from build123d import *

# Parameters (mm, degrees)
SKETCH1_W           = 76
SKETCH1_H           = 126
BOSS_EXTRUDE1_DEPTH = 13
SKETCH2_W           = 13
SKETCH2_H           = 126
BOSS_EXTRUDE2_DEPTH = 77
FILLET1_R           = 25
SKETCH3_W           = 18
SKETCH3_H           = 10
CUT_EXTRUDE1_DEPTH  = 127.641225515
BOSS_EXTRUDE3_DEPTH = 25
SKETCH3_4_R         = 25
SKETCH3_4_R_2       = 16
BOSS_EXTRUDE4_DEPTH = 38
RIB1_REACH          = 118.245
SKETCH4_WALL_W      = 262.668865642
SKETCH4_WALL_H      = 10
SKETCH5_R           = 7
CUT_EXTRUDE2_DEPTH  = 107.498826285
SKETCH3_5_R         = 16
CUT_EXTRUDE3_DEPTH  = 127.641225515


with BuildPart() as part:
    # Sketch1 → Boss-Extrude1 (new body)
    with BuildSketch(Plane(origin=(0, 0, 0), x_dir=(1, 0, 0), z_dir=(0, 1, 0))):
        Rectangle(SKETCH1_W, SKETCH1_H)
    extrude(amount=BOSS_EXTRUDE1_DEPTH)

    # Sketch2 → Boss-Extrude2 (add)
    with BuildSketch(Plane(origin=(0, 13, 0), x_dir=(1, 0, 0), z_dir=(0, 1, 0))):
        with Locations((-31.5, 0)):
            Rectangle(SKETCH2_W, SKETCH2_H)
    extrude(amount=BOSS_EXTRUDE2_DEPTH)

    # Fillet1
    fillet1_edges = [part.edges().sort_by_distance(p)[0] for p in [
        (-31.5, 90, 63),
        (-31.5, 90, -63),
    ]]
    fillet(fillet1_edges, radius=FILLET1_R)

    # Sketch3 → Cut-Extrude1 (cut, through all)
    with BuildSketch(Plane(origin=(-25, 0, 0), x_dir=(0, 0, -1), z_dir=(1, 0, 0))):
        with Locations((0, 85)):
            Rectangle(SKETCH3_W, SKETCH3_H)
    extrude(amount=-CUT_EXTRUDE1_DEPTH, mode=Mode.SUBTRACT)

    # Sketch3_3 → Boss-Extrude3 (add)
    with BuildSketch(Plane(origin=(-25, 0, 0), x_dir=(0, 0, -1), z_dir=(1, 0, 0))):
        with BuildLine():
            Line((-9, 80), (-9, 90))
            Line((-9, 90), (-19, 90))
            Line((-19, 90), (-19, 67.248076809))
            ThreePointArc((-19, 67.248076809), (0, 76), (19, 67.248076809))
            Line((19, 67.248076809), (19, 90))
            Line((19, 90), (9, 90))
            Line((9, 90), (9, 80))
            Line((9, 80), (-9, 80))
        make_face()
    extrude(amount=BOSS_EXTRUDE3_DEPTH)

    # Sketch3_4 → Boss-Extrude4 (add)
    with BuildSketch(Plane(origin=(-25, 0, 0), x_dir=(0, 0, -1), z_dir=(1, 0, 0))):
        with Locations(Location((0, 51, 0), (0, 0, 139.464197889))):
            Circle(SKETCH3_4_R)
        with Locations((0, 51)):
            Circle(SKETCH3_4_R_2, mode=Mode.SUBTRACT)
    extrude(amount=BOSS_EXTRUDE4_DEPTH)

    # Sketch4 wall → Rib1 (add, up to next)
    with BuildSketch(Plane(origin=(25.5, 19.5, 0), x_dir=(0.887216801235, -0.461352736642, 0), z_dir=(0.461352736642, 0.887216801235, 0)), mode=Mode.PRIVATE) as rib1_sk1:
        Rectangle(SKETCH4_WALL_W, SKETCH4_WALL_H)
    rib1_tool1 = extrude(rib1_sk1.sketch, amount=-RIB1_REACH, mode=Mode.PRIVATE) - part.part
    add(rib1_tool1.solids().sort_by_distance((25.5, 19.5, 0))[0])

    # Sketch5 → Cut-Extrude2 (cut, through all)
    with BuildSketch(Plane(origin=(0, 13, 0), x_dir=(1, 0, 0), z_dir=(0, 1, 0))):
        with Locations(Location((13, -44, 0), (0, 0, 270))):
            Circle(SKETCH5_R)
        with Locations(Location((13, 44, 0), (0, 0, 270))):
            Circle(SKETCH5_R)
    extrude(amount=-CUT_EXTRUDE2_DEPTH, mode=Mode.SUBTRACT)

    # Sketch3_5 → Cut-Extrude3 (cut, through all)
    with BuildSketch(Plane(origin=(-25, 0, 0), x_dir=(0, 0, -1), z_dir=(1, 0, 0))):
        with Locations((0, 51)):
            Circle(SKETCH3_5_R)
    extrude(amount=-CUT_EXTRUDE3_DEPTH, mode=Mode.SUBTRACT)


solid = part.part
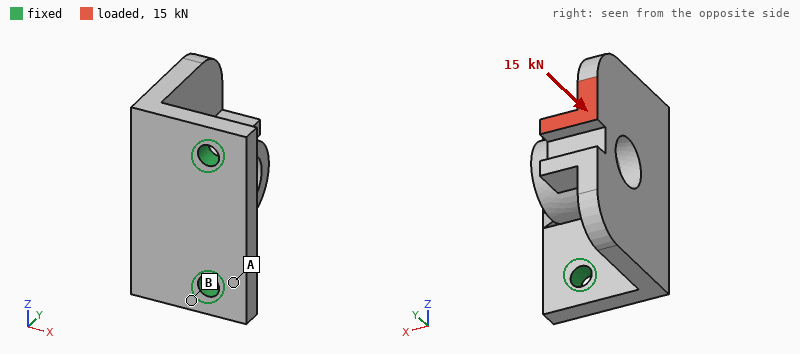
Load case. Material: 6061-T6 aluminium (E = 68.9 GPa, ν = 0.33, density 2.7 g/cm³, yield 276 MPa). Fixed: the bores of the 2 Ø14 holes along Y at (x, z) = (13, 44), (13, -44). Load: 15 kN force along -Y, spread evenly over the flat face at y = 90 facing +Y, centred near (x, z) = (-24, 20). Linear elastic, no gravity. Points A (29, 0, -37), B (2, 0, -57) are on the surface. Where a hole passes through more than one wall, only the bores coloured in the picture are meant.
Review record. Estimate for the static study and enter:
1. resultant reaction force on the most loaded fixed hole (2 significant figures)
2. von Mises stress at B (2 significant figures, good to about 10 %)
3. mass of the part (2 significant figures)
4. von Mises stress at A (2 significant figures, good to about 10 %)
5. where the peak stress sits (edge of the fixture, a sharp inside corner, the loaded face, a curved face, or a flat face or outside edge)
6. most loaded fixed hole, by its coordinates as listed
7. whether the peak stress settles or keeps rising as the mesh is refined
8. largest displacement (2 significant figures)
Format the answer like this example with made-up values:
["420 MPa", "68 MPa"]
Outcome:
["11 kN", "74 MPa", "790 g", "33 MPa", "edge of the fixture", "(13, 44)", "keeps rising", "0.50 mm"]
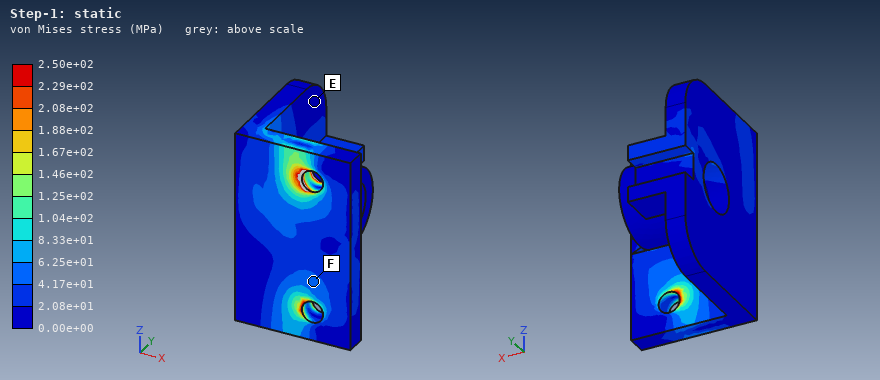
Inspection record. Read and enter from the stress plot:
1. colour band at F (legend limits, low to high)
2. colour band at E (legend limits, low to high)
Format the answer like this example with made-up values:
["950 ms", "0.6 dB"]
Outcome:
["4.17e+01 to 6.25e+01 MPa", "0.00e+00 to 2.08e+01 MPa"]
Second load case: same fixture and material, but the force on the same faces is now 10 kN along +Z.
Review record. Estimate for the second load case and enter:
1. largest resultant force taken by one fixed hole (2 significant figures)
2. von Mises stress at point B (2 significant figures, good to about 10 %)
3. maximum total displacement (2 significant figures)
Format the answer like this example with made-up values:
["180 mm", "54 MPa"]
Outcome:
["11 kN", "93 MPa", "0.36 mm"]
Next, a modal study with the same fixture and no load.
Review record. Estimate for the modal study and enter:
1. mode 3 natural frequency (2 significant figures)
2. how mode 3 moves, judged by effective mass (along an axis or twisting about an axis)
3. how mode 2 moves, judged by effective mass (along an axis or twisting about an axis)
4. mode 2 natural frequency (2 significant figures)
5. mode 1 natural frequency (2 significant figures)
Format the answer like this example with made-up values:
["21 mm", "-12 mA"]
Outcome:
["3300 Hz", "along Y", "along Z", "1900 Hz", "1100 Hz"]
